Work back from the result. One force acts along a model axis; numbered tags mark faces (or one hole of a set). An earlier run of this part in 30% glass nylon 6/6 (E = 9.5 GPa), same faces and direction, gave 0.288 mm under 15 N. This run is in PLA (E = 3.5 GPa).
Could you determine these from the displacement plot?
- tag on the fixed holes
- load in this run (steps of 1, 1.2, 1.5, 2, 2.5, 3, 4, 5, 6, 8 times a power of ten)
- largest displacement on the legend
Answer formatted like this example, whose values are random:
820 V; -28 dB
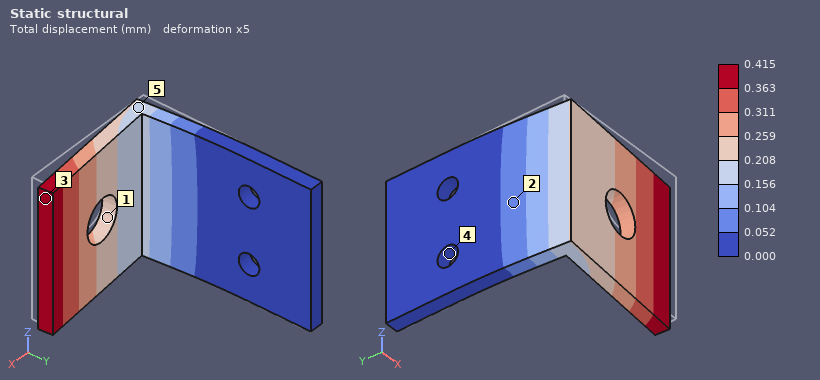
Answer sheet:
4; 8 N; 0.415 mm
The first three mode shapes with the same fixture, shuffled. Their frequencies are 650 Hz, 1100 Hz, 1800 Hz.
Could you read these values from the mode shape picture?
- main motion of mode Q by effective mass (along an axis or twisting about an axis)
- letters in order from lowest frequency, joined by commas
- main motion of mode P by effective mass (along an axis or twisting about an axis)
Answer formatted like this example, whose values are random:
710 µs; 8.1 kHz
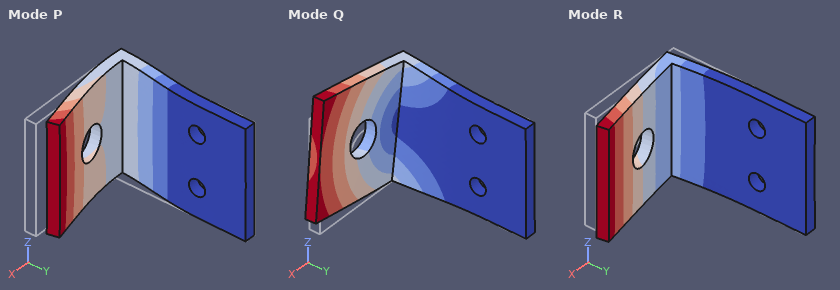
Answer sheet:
along Z; R, Q, P; along X
